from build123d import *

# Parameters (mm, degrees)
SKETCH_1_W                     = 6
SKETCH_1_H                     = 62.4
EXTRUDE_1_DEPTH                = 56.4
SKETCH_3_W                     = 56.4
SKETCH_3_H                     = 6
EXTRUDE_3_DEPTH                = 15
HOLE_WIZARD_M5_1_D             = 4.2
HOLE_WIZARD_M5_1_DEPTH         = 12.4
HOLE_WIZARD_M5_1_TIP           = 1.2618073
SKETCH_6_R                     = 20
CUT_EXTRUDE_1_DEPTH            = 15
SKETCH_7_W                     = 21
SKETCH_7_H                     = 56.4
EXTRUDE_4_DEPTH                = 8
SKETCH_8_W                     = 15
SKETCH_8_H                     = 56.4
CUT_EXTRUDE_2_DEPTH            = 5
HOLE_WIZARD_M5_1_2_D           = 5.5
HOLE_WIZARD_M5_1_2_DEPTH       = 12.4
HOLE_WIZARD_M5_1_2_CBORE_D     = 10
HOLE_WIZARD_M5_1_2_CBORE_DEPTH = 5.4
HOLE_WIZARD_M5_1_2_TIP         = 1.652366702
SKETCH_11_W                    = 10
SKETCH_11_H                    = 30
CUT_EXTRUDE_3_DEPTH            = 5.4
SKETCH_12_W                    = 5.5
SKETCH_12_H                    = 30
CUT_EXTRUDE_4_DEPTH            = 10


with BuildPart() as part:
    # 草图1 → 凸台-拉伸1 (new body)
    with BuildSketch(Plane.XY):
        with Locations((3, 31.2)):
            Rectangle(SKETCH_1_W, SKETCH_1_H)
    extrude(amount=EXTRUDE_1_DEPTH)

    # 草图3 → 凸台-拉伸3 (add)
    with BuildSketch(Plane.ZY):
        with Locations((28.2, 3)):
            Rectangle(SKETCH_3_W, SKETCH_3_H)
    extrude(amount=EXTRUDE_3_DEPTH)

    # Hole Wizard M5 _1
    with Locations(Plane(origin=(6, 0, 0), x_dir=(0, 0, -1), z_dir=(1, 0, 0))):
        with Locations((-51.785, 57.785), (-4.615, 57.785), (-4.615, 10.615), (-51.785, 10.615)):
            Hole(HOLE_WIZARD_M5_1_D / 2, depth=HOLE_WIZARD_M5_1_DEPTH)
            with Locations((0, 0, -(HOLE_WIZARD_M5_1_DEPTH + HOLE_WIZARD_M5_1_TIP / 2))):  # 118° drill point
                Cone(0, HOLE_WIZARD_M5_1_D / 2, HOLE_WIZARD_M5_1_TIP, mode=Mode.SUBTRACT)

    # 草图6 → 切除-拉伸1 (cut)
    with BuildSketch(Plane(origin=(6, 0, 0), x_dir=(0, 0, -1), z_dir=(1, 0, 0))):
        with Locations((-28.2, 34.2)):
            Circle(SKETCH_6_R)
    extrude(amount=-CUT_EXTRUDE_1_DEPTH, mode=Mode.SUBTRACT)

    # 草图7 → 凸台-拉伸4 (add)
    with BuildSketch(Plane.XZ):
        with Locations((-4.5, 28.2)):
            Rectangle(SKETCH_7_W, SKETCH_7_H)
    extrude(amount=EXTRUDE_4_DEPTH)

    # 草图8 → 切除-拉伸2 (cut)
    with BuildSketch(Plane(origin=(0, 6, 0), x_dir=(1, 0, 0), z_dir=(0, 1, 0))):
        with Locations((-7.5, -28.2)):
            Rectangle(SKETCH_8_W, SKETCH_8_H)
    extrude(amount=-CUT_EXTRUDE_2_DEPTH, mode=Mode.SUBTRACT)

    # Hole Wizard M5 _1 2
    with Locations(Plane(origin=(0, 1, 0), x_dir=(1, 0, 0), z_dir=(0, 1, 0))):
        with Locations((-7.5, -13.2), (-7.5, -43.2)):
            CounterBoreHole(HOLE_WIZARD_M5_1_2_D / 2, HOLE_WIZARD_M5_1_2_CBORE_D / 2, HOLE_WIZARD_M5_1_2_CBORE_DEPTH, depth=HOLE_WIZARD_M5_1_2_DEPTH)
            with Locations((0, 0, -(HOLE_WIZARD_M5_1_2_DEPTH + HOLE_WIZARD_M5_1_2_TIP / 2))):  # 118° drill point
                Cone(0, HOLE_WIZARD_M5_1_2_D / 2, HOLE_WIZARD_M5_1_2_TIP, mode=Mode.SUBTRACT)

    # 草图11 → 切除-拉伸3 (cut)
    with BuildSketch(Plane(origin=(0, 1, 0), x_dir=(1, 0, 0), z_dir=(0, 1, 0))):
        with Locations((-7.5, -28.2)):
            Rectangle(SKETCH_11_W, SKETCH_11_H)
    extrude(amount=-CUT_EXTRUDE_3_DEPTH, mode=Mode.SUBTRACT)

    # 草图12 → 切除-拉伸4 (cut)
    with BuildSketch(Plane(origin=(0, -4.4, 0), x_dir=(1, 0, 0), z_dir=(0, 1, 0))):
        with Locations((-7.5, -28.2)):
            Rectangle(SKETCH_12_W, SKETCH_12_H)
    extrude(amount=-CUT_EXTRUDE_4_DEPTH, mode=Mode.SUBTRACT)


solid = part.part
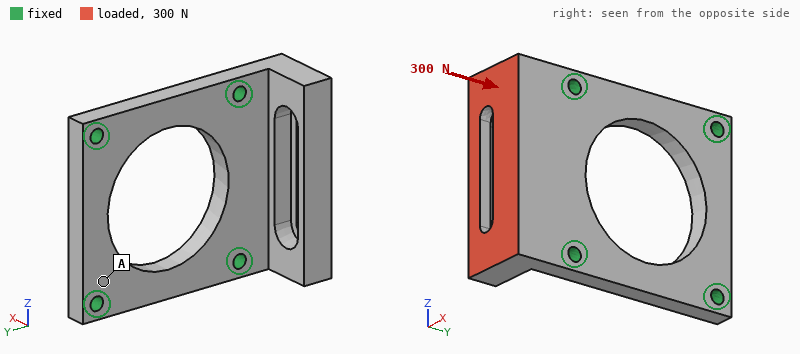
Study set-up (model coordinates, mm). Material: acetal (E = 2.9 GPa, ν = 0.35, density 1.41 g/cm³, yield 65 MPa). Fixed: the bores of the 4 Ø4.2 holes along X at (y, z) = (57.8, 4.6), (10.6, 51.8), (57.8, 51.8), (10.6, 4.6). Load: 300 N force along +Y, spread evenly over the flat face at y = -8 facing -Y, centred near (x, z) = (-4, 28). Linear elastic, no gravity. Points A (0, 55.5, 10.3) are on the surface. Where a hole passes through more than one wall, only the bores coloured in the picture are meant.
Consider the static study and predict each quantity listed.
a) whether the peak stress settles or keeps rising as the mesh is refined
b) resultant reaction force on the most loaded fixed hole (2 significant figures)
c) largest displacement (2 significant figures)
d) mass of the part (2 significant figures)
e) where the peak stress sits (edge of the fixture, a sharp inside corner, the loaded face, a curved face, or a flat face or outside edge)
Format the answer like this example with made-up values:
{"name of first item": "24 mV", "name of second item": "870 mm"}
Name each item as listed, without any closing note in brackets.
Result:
{"whether the peak stress settles or keeps rising as the mesh is refined": "keeps rising", "resultant reaction force on the most loaded fixed hole": "150 N", "largest displacement": "0.36 mm", "mass of the part": "29 g", "where the peak stress sits": "edge of the fixture"}
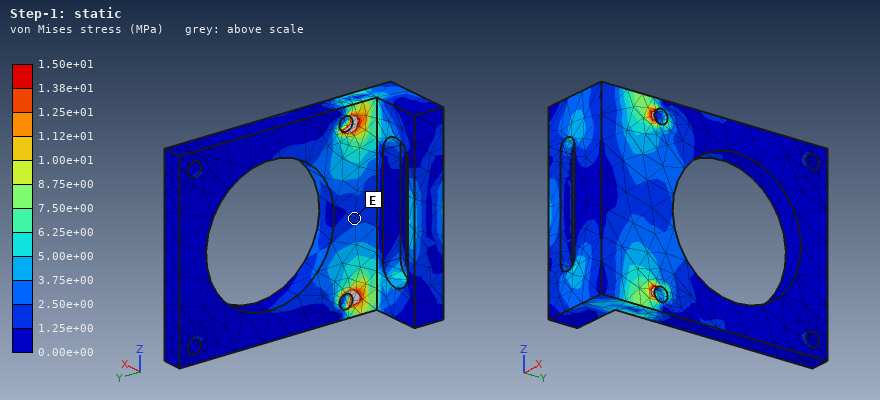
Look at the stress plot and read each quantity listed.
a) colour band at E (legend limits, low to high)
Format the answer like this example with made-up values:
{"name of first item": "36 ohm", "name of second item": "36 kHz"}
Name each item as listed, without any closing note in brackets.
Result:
{"colour band at E": "1.25e+00 to 2.50e+00 MPa"}
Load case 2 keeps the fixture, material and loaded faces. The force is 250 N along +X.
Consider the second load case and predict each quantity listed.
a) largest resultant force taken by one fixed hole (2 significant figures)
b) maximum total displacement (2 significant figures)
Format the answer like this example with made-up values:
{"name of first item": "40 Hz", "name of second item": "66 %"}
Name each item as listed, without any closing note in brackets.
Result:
{"largest resultant force taken by one fixed hole": "130 N", "maximum total displacement": "0.52 mm"}
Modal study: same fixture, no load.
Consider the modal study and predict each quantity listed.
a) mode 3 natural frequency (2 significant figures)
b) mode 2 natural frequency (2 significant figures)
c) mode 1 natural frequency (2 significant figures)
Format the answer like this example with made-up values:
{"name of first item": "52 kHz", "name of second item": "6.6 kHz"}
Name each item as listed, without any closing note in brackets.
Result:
{"mode 3 natural frequency": "3100 Hz", "mode 2 natural frequency": "2400 Hz", "mode 1 natural frequency": "1400 Hz"}
